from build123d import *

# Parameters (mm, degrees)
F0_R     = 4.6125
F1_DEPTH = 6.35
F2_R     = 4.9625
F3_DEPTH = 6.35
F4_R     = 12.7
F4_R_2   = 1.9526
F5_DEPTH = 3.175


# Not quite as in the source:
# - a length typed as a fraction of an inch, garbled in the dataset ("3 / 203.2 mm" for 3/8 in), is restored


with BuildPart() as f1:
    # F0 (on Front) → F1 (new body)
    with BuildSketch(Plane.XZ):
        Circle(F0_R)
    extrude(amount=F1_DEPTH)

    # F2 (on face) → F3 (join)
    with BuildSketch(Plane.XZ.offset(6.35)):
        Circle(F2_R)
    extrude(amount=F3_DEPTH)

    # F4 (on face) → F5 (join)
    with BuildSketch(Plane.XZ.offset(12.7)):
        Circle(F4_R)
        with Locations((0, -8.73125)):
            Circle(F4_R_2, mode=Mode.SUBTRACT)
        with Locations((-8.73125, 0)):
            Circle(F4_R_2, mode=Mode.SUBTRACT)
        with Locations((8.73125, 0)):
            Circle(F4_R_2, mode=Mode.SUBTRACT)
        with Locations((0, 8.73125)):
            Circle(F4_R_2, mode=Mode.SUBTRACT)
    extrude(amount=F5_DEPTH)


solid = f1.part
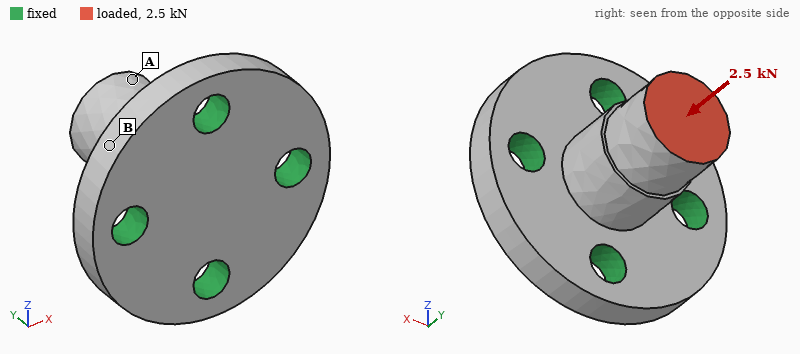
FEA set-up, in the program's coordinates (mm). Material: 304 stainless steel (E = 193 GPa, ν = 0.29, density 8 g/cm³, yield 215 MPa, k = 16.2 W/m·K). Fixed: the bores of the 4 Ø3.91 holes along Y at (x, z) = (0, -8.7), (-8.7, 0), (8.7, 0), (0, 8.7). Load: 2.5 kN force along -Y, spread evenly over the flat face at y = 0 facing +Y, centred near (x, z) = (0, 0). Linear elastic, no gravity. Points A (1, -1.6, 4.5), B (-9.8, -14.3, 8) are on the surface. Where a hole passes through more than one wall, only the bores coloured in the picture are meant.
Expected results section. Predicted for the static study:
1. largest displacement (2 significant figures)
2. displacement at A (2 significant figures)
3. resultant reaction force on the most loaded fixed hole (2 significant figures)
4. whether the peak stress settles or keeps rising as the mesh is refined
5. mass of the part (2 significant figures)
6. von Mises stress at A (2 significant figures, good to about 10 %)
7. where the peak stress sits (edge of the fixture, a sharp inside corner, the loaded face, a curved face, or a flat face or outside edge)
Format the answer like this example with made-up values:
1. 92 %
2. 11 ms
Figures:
1. 4.4 µm
2. 4.1 µm
3. 660 N
4. keeps rising
5. 19 g
6. 37 MPa
7. edge of the fixture
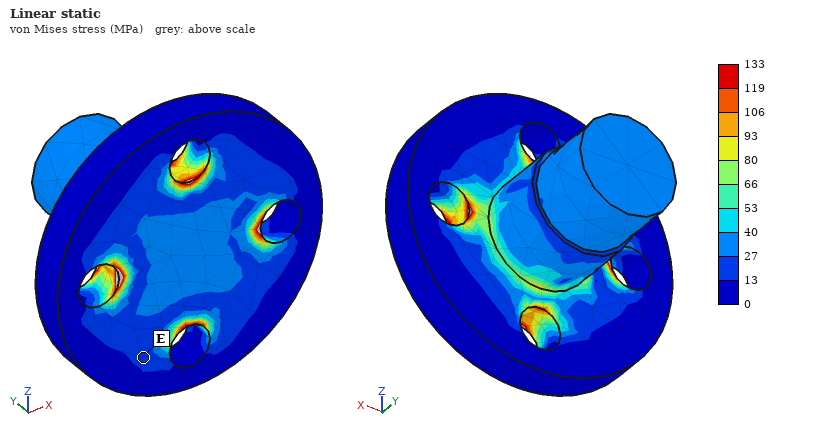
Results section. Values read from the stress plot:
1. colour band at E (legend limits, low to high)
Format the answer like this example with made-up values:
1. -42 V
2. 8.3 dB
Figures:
1. 13 to 27 MPa
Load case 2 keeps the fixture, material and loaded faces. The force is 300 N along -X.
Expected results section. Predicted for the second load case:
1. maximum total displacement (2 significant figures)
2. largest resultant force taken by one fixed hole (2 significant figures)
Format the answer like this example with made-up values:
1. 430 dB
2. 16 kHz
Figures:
1. 5.9 µm
2. 320 N
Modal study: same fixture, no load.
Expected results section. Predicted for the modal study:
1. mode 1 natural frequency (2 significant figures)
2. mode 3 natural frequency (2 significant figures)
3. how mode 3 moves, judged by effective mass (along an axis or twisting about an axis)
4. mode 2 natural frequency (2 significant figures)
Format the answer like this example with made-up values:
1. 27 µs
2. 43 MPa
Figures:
1. 24 kHz
2. 50 kHz
3. along Y
4. 24 kHz
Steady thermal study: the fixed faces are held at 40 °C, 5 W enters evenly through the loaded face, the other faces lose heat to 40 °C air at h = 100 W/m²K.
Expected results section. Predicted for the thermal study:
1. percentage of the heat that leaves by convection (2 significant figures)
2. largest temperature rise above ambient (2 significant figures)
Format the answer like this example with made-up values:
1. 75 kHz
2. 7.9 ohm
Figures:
1. 29 %
2. 58 K
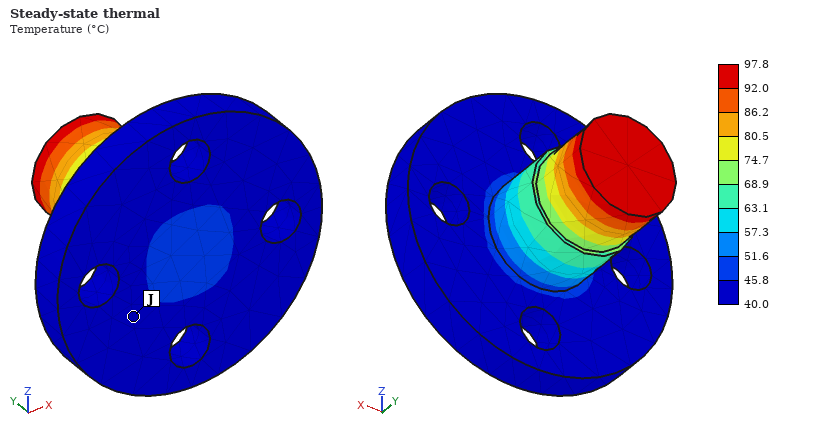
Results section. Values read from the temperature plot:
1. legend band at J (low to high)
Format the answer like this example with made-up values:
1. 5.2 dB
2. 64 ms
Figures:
1. 40.0 to 45.8 °C
